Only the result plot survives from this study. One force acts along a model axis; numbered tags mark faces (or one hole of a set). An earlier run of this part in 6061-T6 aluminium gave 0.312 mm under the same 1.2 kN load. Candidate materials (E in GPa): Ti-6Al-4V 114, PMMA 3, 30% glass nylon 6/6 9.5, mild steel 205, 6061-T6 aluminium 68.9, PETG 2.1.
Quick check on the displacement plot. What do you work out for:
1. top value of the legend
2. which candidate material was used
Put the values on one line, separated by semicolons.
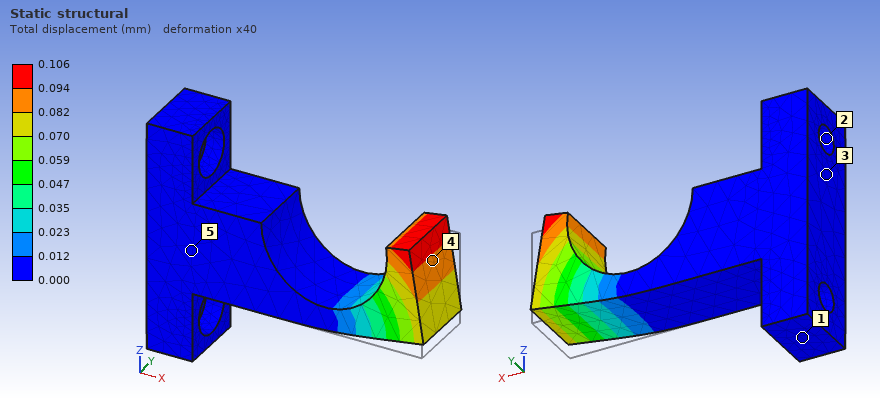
0.106 mm; mild steel
